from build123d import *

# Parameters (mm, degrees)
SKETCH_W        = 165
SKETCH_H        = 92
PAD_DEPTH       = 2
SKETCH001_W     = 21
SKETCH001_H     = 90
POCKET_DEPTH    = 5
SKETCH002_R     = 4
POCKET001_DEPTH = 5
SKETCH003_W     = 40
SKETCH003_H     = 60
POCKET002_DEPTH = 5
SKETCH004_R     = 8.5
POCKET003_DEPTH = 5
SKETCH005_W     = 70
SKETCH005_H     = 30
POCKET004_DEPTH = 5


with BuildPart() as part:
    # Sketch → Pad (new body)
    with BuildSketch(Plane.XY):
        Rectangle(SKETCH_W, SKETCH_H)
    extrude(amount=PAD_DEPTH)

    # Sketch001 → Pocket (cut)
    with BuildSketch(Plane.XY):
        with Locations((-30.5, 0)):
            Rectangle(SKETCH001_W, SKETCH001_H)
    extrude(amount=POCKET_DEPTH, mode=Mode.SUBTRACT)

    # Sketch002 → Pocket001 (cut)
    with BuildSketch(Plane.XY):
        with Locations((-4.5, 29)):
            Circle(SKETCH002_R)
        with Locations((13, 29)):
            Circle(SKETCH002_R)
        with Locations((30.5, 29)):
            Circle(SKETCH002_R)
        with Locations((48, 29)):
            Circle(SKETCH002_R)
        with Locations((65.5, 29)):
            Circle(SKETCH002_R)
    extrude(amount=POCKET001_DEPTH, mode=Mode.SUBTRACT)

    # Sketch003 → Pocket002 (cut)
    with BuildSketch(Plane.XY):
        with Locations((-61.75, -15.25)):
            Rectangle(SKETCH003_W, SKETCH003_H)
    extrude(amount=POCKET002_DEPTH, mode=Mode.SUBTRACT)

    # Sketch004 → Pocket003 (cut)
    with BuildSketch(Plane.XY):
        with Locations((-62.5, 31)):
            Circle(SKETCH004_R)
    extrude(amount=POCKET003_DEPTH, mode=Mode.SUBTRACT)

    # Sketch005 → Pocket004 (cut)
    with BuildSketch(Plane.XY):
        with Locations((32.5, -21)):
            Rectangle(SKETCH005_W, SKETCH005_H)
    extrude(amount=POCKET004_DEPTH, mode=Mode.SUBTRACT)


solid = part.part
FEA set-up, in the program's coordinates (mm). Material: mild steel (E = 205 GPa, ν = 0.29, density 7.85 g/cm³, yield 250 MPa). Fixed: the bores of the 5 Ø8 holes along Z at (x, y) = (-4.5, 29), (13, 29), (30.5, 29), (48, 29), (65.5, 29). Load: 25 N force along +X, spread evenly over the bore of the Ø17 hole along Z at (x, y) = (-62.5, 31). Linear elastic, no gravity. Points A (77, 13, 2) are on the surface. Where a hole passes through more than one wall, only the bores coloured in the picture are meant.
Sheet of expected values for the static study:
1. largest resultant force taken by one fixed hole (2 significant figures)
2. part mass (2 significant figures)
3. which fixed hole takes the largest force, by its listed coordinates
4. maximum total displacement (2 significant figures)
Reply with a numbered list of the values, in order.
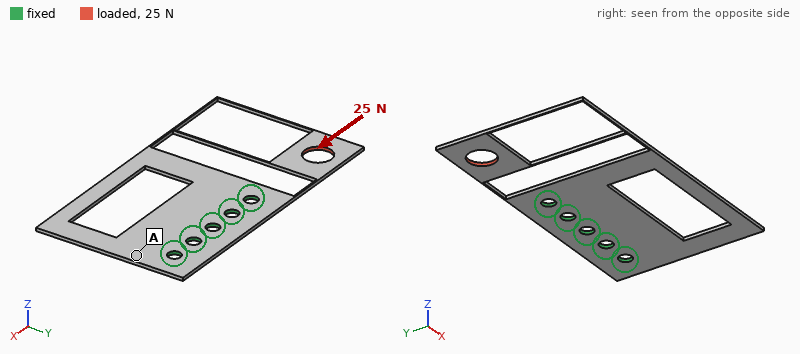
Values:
1. 13 N
2. 130 g
3. (-4.5, 29)
4. 1.7 mm
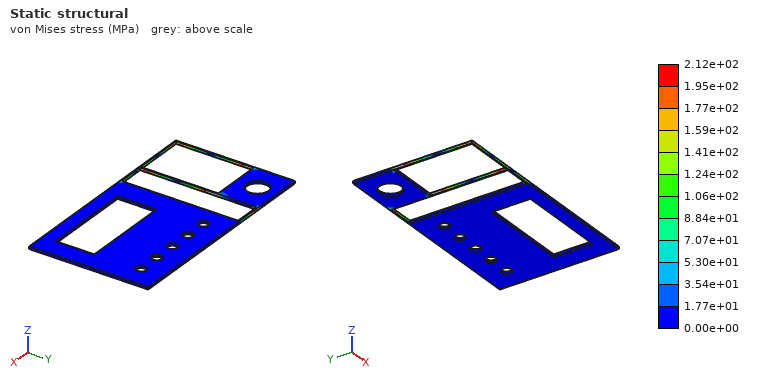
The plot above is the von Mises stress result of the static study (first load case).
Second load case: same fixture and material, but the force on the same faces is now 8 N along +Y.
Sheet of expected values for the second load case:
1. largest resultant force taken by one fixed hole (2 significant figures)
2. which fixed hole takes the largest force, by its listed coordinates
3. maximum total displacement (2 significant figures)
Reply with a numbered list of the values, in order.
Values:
1. 14 N
2. (-4.5, 29)
3. 1.2 mm
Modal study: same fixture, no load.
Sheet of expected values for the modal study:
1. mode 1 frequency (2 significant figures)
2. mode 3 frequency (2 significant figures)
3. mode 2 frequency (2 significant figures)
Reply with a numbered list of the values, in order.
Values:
1. 93 Hz
2. 280 Hz
3. 110 Hz
